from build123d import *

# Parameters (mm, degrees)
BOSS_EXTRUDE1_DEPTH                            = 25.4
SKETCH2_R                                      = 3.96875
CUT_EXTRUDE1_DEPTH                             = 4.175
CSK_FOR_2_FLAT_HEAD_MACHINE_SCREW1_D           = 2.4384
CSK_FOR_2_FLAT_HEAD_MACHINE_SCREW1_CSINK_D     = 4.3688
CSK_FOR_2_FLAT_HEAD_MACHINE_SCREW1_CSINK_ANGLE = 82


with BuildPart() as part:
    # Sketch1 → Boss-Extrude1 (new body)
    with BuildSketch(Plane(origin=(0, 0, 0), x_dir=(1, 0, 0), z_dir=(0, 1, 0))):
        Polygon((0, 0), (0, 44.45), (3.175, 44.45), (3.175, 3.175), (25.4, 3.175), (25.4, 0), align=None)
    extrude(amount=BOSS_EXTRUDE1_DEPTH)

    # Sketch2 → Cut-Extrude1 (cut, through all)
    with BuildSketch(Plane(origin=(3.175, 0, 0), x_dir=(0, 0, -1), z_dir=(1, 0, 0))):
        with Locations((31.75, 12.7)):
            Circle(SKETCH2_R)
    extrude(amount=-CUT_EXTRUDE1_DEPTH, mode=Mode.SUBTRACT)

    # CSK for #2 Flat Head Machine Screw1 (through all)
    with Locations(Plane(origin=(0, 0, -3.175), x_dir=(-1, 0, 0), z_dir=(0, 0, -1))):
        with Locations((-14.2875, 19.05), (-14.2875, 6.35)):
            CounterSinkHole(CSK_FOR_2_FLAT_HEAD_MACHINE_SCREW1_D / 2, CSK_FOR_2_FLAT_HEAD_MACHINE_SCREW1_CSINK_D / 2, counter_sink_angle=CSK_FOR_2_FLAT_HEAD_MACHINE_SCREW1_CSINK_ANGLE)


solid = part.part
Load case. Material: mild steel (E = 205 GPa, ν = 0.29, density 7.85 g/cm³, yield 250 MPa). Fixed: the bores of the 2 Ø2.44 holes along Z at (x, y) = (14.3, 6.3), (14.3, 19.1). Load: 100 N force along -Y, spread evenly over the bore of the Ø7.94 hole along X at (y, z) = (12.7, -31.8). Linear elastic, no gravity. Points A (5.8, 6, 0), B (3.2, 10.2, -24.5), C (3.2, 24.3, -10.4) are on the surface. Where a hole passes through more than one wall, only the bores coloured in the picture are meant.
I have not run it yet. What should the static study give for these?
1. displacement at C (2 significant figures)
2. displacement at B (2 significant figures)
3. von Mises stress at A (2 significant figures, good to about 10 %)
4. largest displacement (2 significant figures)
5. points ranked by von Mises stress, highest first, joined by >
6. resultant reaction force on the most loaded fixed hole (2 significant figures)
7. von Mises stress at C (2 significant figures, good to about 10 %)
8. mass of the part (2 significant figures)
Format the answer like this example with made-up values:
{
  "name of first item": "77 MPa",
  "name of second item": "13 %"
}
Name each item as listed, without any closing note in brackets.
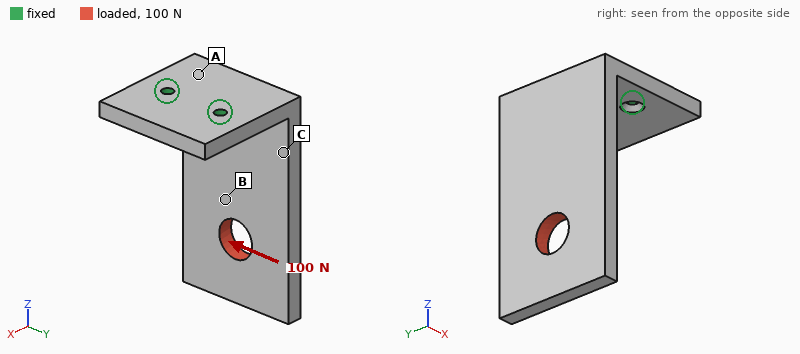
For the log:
{
  "displacement at C": "15 µm",
  "displacement at B": "24 µm",
  "von Mises stress at A": "31 MPa",
  "largest displacement": "47 µm",
  "points ranked by von Mises stress, highest first, joined by >": "A > C > B",
  "resultant reaction force on the most loaded fixed hole": "230 N",
  "von Mises stress at C": "16 MPa",
  "mass of the part": "41 g"
}
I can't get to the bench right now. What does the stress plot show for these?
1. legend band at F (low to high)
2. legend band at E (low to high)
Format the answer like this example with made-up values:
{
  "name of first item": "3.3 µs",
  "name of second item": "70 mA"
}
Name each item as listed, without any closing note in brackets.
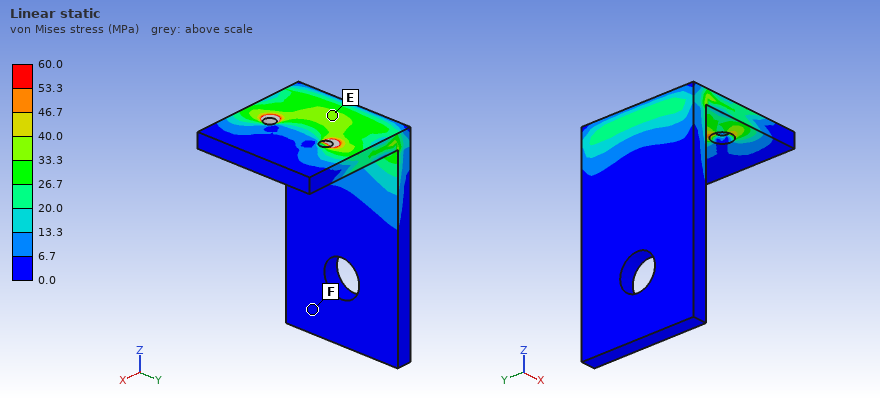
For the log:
{
  "legend band at F": "0.0 to 6.7 MPa",
  "legend band at E": "33.3 to 40.0 MPa"
}
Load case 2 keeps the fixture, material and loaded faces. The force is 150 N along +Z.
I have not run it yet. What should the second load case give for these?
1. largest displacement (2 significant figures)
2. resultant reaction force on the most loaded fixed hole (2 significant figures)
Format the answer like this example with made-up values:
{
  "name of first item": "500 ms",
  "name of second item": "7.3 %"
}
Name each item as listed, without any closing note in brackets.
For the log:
{
  "largest displacement": "51 µm",
  "resultant reaction force on the most loaded fixed hole": "75 N"
}
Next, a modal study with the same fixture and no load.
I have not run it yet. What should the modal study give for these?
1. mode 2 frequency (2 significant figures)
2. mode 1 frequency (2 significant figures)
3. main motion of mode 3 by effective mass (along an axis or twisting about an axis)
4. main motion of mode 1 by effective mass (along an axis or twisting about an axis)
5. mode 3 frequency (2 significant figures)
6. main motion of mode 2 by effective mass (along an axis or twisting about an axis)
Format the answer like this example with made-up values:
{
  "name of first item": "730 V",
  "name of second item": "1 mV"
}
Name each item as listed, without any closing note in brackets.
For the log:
{
  "mode 2 frequency": "2100 Hz",
  "mode 1 frequency": "970 Hz",
  "main motion of mode 3 by effective mass": "along Z",
  "main motion of mode 1 by effective mass": "along X",
  "mode 3 frequency": "4400 Hz",
  "main motion of mode 2 by effective mass": "along Y"
}
